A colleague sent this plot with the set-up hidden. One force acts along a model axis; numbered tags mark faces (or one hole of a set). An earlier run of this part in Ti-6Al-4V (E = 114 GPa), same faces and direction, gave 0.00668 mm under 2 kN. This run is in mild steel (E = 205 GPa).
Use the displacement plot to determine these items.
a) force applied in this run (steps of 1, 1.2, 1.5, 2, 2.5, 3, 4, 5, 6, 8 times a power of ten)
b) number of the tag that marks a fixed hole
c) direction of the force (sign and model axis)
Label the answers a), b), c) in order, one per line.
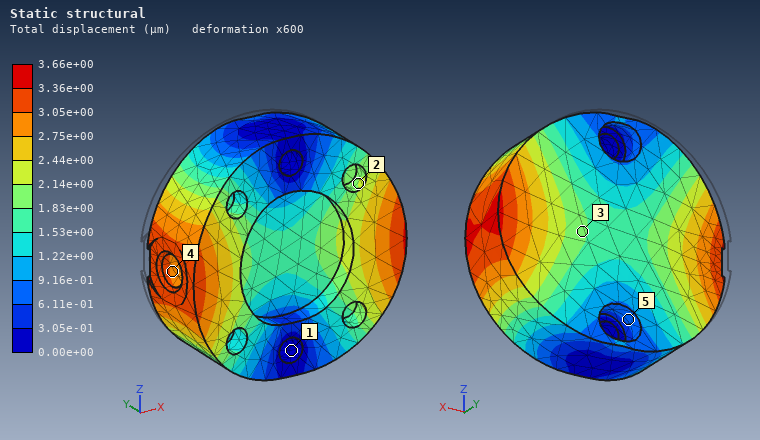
a) 2 kN
b) 1
c) -Y
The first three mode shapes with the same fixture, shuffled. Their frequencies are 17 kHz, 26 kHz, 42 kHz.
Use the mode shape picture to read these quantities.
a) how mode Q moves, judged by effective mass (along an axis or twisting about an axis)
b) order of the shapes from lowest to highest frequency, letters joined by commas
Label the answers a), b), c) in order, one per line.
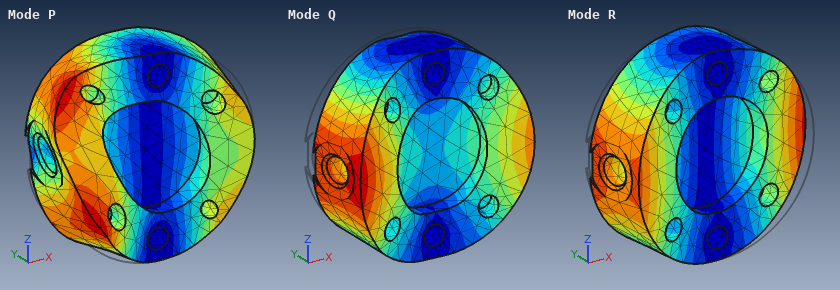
a) along Y
b) R, Q, P
